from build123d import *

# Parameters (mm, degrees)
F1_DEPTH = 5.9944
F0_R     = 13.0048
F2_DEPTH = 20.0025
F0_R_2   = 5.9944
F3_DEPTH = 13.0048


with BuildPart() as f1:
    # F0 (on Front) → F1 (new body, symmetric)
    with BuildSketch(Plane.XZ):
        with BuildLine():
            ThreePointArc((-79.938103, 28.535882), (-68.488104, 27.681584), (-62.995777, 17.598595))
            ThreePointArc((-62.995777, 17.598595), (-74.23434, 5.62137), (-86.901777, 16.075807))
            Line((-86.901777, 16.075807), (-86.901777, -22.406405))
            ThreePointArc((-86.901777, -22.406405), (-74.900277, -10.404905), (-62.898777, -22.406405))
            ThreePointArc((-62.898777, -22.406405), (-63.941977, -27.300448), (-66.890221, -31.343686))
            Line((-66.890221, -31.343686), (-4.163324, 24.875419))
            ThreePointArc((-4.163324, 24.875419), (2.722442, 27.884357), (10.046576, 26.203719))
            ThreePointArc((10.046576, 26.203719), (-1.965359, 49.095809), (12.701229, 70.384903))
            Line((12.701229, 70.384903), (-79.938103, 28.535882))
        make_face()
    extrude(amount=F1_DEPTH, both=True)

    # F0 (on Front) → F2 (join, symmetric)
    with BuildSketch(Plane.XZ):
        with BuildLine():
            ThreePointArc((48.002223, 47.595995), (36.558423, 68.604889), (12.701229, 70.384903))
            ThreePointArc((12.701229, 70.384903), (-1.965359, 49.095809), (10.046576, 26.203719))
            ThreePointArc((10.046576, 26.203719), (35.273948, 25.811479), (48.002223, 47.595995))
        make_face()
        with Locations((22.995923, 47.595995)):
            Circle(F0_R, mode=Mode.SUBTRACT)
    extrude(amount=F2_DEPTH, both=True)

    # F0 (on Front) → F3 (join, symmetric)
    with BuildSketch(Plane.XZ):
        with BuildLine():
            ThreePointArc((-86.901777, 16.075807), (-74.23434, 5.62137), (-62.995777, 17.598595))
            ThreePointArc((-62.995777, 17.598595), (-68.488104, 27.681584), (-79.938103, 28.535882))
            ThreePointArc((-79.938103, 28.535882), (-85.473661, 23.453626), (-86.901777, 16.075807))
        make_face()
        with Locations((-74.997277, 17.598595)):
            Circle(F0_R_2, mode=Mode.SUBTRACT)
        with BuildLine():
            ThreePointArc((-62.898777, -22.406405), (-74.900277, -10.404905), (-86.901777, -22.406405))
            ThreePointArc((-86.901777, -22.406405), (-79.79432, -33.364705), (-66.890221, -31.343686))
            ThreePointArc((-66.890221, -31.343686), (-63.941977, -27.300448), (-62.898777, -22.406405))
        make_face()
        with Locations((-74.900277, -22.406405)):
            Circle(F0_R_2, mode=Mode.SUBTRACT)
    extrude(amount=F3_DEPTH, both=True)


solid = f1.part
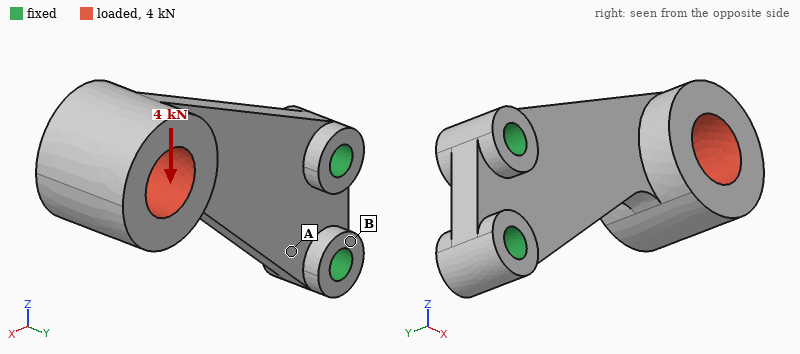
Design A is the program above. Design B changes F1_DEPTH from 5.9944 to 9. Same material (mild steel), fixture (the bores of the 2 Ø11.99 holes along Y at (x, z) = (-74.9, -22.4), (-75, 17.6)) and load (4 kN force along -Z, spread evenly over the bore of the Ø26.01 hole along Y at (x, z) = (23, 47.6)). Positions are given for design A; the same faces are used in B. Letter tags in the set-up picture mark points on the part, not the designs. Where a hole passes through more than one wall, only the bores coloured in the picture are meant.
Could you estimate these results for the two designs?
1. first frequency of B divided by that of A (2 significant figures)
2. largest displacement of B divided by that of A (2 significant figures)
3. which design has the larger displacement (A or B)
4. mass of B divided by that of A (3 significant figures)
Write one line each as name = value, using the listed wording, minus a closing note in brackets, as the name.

first frequency of B divided by that of A = 1.7
largest displacement of B divided by that of A = 0.69
which design has the larger displacement = A
mass of B divided by that of A = 1.19
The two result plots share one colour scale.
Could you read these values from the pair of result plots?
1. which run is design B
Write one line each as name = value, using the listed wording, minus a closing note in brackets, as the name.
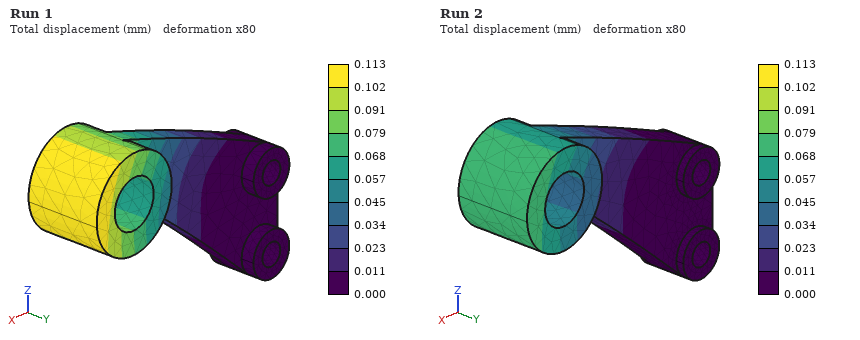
which run is design B = Run 2
